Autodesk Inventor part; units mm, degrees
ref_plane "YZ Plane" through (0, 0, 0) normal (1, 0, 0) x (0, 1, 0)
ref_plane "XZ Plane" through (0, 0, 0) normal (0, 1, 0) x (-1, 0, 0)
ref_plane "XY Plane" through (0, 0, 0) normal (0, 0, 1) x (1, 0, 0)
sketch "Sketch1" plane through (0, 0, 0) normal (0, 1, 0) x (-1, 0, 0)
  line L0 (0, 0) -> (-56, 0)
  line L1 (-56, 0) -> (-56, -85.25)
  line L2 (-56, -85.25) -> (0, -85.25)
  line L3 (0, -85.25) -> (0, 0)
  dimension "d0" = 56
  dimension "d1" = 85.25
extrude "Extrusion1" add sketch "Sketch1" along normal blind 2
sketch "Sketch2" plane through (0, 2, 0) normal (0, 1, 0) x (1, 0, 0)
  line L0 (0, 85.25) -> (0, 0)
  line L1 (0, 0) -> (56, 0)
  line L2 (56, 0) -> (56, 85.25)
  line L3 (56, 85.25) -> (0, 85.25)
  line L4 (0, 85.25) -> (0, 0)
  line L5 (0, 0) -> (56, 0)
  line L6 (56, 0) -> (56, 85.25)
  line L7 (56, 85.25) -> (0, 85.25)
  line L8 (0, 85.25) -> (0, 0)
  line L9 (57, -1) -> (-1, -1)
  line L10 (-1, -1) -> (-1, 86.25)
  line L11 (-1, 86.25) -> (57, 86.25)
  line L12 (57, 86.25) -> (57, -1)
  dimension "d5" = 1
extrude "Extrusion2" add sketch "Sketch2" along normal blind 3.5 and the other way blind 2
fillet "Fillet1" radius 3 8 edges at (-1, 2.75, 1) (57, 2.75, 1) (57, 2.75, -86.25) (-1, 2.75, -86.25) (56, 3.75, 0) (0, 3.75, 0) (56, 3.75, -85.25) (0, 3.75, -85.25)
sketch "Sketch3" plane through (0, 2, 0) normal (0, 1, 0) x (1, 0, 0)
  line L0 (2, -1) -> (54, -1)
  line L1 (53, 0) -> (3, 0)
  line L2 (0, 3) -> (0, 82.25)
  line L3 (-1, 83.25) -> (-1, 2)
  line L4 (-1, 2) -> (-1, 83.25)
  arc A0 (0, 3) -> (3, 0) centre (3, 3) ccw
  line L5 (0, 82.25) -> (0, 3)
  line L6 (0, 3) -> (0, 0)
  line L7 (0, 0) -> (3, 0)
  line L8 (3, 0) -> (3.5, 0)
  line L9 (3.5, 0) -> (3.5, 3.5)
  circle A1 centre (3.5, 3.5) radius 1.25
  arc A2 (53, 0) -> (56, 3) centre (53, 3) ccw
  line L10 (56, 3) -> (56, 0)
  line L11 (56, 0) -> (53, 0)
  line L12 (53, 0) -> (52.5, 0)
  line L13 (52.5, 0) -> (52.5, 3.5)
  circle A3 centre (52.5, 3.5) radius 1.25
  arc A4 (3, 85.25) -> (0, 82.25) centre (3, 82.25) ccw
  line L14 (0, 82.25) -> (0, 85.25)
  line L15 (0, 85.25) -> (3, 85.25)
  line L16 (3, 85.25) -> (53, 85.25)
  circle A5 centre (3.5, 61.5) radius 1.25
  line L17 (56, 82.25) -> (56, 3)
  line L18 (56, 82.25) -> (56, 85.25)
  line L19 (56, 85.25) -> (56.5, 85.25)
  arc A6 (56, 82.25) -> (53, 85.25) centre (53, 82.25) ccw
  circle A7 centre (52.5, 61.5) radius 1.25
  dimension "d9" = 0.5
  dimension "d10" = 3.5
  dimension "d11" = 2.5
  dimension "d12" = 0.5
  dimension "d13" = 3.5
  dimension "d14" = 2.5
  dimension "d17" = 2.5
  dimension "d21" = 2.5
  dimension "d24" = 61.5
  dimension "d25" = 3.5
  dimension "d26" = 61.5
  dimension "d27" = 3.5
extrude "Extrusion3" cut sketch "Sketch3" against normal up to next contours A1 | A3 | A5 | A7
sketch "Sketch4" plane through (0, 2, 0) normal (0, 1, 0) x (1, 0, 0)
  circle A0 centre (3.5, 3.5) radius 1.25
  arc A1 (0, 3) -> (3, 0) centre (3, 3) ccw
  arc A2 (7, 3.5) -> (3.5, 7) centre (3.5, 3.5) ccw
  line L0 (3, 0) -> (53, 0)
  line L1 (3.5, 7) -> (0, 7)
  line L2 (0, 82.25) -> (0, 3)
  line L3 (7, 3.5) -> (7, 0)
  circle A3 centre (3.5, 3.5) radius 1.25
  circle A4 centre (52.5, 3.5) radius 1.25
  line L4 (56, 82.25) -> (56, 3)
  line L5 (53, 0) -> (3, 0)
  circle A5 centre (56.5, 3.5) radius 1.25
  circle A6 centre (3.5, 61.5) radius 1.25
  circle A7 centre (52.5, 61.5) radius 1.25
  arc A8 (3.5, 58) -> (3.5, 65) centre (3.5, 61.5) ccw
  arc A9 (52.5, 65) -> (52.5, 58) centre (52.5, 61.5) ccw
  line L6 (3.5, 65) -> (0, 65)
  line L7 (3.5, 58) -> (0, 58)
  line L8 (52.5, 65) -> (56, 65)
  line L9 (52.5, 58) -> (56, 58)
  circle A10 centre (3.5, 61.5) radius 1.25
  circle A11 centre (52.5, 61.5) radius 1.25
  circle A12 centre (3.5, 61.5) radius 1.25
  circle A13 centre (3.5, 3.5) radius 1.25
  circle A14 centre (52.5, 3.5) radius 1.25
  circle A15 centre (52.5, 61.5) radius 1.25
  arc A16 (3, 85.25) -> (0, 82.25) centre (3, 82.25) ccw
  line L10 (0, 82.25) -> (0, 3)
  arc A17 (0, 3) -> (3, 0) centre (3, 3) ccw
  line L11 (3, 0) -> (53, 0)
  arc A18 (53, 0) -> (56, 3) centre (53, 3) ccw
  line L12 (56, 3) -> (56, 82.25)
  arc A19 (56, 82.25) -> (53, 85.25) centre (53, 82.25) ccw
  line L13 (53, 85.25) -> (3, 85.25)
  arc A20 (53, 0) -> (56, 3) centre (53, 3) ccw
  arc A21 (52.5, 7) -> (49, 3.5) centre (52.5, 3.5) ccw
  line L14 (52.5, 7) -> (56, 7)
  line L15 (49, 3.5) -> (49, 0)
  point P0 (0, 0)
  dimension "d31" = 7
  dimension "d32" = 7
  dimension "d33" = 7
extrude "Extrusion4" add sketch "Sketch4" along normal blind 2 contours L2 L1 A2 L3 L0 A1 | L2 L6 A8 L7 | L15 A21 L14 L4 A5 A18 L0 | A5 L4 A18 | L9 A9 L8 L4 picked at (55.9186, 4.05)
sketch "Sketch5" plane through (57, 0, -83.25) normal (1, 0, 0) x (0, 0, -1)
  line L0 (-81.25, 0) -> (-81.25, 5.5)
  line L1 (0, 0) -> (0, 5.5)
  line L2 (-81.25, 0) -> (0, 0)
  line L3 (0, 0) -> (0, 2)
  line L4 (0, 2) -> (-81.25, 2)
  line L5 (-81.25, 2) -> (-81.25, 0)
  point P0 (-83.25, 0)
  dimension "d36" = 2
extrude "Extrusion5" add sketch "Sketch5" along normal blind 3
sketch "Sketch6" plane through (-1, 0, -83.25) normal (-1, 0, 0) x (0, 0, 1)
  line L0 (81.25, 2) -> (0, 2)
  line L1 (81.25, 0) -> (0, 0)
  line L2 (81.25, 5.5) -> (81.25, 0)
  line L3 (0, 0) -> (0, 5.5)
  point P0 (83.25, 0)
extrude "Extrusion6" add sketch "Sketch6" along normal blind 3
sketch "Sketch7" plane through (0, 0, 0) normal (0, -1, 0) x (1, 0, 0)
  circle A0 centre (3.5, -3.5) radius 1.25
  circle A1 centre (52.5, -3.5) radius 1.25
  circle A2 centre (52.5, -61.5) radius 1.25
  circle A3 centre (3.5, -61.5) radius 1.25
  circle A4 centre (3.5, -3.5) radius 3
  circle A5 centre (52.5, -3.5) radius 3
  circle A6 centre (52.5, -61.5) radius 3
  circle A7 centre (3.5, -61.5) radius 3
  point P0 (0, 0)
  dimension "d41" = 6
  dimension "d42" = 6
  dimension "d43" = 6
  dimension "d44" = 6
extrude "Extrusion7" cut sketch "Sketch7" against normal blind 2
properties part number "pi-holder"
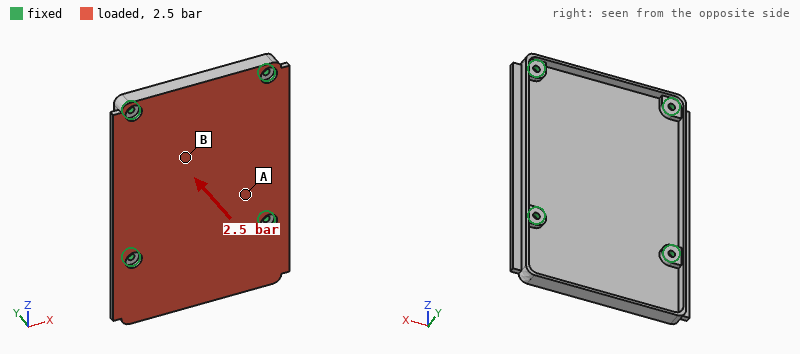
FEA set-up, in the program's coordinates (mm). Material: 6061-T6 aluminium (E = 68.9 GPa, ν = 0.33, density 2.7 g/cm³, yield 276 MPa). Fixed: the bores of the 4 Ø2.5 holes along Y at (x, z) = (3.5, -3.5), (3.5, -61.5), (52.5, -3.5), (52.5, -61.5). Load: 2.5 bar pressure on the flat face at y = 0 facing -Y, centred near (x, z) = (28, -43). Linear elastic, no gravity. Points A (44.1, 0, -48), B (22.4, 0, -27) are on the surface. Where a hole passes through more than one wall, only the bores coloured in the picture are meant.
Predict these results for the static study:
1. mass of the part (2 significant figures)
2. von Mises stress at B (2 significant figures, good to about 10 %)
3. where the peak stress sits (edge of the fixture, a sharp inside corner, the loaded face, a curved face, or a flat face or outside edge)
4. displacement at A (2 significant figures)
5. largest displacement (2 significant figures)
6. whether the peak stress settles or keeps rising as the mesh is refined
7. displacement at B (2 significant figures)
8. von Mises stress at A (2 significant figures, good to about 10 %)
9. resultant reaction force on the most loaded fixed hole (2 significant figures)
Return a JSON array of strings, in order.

["33 g", "52 MPa", "edge of the fixture", "0.11 mm", "0.22 mm", "keeps rising", "0.21 mm", "17 MPa", "660 N"]
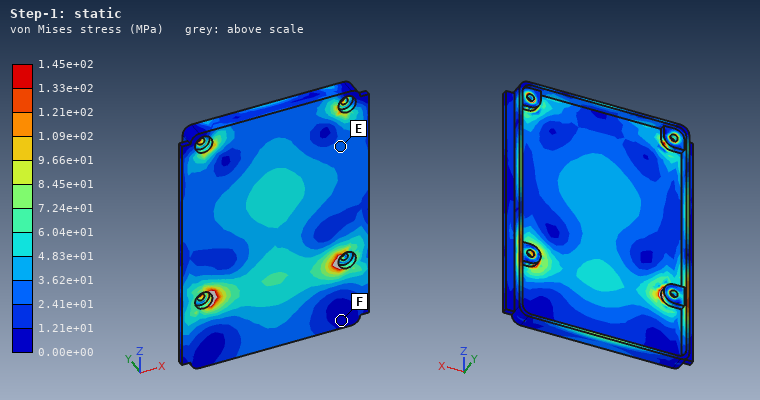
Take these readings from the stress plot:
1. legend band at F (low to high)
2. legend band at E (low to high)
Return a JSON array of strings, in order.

["0.00e+00 to 1.21e+01 MPa", "2.41e+01 to 3.62e+01 MPa"]
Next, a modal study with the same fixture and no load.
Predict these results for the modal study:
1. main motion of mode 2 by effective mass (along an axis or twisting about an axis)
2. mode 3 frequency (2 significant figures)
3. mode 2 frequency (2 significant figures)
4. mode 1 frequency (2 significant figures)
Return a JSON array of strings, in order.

["along Y", "4100 Hz", "2800 Hz", "2400 Hz"]
